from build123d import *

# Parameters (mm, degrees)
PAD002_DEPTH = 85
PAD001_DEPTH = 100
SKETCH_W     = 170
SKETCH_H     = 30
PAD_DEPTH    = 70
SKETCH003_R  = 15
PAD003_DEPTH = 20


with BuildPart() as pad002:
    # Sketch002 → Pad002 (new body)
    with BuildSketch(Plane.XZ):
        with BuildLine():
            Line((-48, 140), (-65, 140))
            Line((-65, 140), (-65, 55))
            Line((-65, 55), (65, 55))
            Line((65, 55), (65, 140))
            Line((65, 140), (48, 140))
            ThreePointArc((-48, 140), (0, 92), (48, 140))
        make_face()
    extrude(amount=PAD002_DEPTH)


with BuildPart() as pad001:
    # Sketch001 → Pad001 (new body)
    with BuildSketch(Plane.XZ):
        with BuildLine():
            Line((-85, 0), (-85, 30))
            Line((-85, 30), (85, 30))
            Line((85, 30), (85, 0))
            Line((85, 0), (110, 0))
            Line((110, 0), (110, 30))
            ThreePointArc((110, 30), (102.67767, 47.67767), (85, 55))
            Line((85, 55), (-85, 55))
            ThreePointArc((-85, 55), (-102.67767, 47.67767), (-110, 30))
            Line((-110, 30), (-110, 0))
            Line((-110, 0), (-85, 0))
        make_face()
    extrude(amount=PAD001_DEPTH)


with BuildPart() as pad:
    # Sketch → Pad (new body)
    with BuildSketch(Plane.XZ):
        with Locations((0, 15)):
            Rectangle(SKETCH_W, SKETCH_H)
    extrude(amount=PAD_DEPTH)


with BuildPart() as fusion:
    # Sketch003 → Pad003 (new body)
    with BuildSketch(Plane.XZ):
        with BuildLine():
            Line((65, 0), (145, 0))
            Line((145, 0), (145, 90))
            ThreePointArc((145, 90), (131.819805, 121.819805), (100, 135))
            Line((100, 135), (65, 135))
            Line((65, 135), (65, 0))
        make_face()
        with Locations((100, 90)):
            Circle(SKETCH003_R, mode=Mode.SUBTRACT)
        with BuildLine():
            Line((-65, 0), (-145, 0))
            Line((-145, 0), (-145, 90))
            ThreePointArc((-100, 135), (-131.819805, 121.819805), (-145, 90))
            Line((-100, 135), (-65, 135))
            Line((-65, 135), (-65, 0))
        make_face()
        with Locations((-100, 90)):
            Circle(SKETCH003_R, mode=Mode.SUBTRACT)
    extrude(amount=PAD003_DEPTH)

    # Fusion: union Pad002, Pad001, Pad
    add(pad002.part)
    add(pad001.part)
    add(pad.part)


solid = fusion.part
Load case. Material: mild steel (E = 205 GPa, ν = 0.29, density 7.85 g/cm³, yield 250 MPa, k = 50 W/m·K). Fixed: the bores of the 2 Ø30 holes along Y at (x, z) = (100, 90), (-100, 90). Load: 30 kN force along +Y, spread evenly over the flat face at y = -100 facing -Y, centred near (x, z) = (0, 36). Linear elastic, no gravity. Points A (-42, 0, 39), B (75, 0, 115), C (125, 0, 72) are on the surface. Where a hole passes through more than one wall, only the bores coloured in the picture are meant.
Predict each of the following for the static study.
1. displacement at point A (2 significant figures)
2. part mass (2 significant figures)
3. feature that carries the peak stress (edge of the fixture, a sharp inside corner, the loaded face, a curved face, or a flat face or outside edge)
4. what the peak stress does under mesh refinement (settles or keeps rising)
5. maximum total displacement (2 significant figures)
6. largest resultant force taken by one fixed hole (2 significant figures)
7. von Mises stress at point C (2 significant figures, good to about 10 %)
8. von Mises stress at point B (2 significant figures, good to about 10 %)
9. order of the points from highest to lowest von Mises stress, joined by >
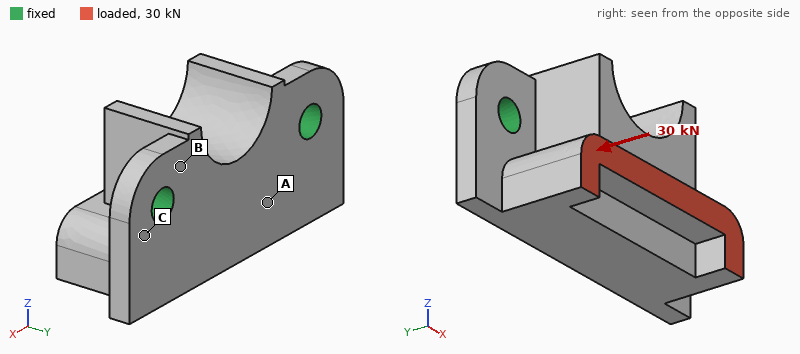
33 µm
15 kg
edge of the fixture
keeps rising
79 µm
15 kN
37 MPa
25 MPa
C > B > A
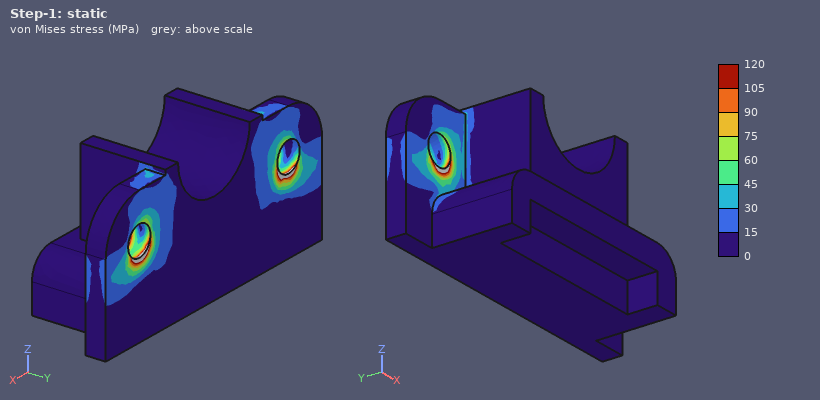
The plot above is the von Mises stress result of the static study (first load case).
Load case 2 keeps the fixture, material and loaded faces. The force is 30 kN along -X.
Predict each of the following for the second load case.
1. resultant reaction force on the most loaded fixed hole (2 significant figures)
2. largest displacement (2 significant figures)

23 kN
25 µm
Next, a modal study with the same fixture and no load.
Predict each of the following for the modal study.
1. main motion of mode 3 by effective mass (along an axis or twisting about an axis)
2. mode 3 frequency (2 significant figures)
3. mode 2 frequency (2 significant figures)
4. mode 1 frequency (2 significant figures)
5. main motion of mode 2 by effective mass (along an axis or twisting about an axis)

along Y
2900 Hz
2800 Hz
1000 Hz
along X
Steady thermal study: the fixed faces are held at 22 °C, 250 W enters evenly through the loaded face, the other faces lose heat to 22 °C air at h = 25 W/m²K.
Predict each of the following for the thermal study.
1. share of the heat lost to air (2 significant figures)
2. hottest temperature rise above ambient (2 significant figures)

39 %
69 K
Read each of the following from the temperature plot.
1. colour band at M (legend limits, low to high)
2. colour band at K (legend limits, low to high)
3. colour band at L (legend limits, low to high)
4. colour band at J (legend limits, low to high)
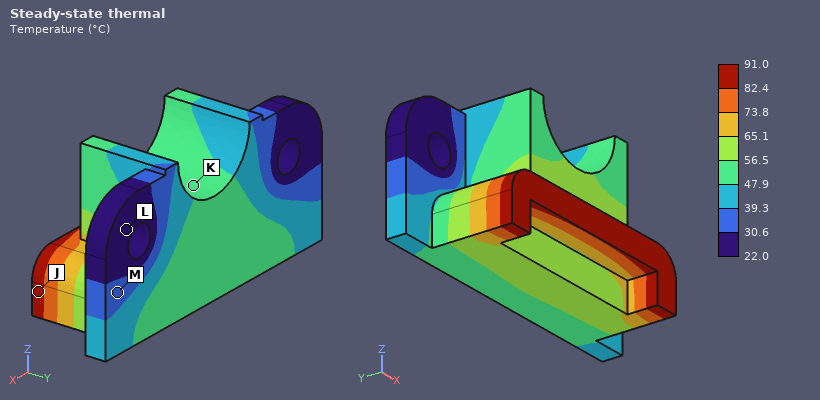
30.6 to 39.3 °C
47.9 to 56.5 °C
22.0 to 30.6 °C
82.4 to 91.0 °C
